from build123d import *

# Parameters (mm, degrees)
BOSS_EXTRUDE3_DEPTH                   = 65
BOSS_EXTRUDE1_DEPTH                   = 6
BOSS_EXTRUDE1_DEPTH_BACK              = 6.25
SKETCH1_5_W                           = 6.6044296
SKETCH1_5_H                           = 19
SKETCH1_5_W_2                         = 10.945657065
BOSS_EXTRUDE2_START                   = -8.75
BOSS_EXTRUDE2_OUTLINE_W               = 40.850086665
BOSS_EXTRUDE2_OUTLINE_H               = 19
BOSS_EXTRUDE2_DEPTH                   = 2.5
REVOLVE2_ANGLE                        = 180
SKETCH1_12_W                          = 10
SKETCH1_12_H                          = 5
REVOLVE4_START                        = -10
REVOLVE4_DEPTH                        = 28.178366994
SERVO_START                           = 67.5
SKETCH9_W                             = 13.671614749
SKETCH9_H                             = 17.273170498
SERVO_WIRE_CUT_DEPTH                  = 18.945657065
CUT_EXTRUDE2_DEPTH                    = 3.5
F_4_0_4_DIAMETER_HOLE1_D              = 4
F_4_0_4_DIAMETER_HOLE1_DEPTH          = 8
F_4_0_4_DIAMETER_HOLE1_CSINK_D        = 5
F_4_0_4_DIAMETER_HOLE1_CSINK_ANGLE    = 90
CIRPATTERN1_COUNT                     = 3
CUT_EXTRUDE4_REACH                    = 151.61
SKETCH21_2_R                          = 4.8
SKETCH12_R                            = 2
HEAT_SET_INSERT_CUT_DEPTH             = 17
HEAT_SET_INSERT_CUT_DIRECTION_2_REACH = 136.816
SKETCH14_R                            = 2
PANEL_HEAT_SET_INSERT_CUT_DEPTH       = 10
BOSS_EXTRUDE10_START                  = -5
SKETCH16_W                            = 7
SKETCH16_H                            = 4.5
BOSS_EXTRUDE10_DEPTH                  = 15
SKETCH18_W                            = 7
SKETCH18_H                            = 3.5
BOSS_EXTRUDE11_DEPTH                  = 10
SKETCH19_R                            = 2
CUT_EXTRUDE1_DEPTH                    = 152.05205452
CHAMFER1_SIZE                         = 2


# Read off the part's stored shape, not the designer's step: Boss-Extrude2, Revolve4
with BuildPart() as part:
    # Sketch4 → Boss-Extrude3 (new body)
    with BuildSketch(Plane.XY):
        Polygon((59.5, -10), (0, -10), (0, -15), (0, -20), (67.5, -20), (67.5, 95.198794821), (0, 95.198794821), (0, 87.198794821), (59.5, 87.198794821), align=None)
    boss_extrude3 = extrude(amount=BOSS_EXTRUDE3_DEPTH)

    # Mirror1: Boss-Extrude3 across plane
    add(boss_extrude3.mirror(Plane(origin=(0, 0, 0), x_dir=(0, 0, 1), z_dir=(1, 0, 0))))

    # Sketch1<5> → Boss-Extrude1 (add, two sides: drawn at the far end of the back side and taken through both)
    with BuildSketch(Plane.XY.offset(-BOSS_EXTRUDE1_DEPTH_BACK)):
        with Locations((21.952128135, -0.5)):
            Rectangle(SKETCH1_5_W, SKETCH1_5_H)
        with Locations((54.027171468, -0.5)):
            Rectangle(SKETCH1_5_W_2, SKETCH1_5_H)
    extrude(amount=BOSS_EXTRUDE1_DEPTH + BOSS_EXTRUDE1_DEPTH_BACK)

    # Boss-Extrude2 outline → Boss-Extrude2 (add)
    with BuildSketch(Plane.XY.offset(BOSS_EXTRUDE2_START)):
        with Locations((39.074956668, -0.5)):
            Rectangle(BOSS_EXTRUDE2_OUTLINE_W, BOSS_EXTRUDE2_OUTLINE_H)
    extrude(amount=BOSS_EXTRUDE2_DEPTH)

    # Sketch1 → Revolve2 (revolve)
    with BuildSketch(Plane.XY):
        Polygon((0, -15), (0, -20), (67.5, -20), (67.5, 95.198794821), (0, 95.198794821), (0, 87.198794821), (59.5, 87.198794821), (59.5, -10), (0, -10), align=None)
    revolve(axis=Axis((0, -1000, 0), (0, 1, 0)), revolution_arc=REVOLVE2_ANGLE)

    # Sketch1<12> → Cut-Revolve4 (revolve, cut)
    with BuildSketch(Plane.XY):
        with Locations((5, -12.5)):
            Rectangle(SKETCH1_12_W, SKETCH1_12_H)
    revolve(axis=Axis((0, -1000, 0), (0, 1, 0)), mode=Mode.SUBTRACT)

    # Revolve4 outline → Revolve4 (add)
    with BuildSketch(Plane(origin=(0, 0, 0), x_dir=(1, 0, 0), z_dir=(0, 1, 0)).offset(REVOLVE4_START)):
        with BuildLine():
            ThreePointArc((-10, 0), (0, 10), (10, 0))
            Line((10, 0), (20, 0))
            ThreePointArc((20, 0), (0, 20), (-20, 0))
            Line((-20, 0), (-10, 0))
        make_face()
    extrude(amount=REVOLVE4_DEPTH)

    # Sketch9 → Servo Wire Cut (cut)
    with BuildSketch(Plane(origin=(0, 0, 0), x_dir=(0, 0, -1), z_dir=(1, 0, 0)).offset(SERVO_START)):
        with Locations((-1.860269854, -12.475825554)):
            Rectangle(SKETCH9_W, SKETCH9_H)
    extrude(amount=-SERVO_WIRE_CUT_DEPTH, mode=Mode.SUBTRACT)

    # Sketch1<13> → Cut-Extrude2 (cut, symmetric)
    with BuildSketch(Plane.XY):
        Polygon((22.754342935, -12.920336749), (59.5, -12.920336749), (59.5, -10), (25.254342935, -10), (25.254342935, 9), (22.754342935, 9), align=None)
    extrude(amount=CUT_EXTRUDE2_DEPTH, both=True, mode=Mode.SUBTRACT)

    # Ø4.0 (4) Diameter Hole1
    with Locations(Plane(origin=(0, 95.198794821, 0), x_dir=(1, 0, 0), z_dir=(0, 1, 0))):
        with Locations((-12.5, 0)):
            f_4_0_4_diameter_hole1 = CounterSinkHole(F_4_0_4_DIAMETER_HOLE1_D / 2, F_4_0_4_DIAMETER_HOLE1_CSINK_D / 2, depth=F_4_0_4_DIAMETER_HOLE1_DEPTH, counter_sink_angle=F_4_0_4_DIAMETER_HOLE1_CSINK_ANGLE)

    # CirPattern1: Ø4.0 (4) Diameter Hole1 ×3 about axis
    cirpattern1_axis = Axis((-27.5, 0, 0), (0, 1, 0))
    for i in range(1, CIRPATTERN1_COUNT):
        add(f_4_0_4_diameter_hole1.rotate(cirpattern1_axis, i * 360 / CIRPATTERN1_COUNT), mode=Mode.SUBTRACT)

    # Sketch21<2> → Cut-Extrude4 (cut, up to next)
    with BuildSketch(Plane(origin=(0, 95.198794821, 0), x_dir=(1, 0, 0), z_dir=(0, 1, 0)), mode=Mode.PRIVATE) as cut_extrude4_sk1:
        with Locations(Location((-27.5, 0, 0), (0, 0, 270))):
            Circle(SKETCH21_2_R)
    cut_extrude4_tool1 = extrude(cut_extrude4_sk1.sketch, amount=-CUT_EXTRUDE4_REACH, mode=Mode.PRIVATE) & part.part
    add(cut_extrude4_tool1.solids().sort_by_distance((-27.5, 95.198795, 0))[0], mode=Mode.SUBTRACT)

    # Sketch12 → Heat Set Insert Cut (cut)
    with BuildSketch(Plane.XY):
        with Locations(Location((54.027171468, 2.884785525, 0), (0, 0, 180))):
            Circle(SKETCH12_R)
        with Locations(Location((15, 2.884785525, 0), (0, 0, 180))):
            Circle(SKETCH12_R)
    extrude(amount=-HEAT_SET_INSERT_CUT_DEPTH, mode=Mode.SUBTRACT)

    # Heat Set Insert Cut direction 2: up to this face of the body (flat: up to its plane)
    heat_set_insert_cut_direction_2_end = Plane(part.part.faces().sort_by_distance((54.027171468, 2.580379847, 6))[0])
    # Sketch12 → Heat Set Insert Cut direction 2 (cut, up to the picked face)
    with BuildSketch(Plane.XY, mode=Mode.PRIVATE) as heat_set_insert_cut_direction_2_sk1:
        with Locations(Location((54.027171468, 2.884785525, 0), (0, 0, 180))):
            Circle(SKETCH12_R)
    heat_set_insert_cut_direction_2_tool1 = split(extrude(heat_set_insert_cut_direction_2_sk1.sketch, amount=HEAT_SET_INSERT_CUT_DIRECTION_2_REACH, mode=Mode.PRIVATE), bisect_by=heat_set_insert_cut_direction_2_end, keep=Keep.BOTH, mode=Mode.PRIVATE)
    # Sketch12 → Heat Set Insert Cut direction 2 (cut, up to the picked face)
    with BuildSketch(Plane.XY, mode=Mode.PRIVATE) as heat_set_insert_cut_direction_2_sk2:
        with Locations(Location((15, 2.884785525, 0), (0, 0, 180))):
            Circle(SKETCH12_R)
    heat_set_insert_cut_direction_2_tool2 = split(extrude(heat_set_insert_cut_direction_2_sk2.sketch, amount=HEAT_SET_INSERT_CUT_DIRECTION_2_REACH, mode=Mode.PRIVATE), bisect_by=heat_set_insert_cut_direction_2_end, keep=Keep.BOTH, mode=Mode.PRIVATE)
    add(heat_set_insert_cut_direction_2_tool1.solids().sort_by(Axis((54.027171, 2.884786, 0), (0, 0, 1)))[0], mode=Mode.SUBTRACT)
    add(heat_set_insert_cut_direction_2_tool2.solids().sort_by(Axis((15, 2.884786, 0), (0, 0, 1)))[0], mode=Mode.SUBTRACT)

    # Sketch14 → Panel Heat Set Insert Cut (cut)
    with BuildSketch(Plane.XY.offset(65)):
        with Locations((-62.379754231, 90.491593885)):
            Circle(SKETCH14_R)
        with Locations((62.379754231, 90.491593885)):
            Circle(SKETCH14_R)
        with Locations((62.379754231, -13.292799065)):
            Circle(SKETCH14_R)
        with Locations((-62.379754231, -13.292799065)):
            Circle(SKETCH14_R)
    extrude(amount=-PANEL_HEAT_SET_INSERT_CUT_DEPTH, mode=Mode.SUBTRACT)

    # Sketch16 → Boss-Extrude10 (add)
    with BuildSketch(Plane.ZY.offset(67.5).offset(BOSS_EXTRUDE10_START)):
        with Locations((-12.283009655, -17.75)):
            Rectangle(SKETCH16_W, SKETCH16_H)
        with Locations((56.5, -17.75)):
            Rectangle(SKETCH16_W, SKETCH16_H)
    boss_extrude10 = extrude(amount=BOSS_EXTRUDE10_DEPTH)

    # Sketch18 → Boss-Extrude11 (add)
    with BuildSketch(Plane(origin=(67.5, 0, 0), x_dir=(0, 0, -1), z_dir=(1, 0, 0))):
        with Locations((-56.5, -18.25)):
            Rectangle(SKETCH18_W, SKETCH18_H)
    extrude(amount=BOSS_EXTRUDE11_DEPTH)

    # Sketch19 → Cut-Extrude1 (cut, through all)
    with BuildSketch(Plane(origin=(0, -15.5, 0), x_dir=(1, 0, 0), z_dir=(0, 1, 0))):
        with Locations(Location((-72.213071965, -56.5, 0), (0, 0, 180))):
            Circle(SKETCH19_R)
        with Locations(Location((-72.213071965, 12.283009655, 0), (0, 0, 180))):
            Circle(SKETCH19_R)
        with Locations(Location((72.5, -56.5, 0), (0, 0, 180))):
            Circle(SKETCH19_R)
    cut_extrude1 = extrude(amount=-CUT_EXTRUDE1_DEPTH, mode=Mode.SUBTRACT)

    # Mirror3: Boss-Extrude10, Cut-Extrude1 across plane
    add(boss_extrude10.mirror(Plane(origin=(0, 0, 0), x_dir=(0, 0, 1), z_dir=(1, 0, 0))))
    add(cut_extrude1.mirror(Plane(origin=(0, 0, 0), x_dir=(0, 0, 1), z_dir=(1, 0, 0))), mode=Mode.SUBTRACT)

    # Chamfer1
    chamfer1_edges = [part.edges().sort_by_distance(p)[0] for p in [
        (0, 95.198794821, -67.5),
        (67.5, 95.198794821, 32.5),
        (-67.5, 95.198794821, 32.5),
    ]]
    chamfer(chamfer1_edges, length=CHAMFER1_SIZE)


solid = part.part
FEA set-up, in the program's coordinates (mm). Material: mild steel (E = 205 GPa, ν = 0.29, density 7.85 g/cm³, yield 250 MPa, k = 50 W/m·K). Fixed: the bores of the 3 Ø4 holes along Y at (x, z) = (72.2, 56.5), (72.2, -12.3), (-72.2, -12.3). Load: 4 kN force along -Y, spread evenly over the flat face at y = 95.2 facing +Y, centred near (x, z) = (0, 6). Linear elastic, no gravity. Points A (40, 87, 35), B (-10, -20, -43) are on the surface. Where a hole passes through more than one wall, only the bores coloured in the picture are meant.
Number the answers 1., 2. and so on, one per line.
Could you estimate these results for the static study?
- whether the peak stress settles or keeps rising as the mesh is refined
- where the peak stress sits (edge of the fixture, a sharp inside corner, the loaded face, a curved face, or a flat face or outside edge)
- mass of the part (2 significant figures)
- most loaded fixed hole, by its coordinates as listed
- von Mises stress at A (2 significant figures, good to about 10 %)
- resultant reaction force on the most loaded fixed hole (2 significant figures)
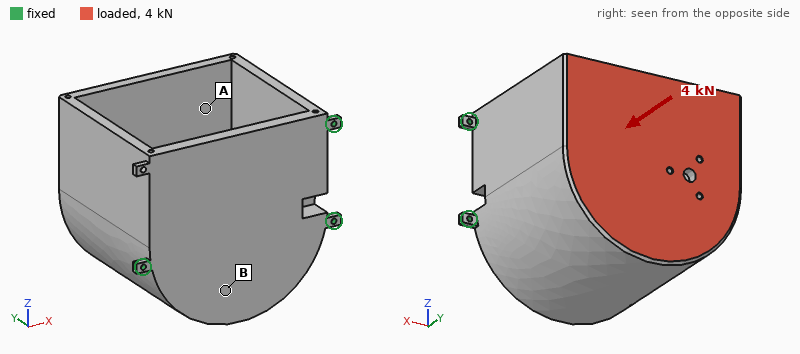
1. keeps rising
2. edge of the fixture
3. 4.4 kg
4. (-72.2, -12.3)
5. 6.6 MPa
6. 2.1 kN
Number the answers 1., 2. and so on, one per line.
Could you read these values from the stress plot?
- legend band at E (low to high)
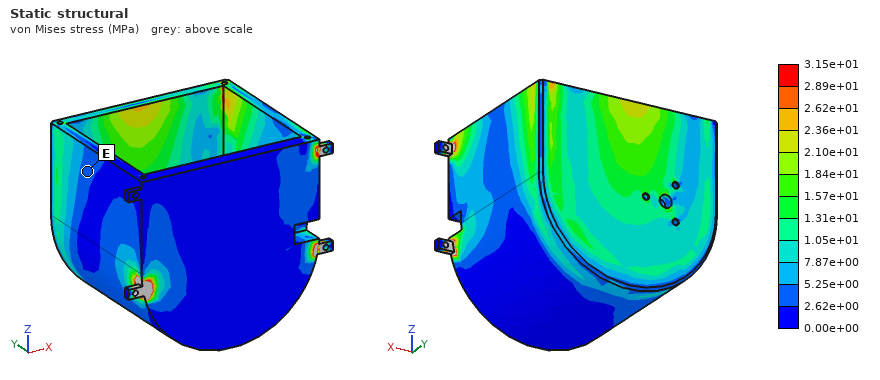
1. 2.62e+00 to 5.25e+00 MPa
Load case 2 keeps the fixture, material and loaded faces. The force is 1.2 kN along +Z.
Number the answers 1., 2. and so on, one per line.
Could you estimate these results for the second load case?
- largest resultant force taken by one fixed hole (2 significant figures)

1. 2.2 kN
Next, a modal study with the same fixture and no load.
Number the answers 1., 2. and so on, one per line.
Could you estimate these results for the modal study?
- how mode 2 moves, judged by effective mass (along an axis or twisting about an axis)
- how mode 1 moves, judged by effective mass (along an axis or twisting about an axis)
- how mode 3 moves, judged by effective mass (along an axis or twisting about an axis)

1. along X
2. along Z
3. along Y
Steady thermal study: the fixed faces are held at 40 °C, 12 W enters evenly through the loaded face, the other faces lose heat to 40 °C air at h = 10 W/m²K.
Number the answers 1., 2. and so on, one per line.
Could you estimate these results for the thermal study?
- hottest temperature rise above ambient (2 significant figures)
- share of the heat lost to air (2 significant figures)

1. 14 K
2. 75 %
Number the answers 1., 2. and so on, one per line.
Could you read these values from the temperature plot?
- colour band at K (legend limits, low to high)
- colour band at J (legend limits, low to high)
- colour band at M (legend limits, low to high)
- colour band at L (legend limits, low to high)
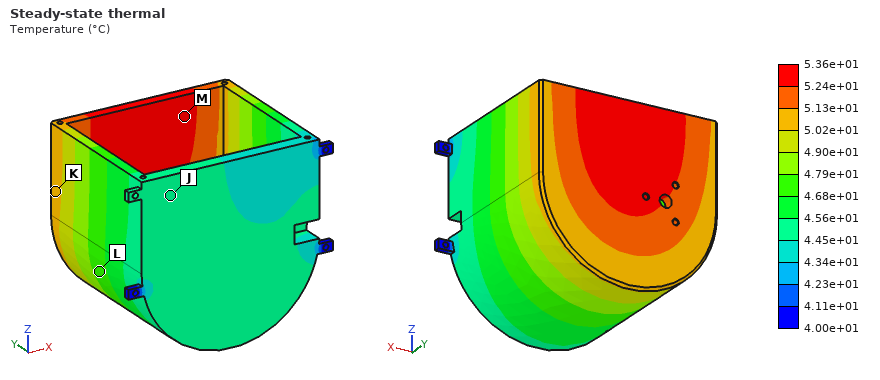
1. 5.02e+01 to 5.13e+01 °C
2. 4.45e+01 to 4.56e+01 °C
3. 5.24e+01 to 5.36e+01 °C
4. 4.68e+01 to 4.79e+01 °C
